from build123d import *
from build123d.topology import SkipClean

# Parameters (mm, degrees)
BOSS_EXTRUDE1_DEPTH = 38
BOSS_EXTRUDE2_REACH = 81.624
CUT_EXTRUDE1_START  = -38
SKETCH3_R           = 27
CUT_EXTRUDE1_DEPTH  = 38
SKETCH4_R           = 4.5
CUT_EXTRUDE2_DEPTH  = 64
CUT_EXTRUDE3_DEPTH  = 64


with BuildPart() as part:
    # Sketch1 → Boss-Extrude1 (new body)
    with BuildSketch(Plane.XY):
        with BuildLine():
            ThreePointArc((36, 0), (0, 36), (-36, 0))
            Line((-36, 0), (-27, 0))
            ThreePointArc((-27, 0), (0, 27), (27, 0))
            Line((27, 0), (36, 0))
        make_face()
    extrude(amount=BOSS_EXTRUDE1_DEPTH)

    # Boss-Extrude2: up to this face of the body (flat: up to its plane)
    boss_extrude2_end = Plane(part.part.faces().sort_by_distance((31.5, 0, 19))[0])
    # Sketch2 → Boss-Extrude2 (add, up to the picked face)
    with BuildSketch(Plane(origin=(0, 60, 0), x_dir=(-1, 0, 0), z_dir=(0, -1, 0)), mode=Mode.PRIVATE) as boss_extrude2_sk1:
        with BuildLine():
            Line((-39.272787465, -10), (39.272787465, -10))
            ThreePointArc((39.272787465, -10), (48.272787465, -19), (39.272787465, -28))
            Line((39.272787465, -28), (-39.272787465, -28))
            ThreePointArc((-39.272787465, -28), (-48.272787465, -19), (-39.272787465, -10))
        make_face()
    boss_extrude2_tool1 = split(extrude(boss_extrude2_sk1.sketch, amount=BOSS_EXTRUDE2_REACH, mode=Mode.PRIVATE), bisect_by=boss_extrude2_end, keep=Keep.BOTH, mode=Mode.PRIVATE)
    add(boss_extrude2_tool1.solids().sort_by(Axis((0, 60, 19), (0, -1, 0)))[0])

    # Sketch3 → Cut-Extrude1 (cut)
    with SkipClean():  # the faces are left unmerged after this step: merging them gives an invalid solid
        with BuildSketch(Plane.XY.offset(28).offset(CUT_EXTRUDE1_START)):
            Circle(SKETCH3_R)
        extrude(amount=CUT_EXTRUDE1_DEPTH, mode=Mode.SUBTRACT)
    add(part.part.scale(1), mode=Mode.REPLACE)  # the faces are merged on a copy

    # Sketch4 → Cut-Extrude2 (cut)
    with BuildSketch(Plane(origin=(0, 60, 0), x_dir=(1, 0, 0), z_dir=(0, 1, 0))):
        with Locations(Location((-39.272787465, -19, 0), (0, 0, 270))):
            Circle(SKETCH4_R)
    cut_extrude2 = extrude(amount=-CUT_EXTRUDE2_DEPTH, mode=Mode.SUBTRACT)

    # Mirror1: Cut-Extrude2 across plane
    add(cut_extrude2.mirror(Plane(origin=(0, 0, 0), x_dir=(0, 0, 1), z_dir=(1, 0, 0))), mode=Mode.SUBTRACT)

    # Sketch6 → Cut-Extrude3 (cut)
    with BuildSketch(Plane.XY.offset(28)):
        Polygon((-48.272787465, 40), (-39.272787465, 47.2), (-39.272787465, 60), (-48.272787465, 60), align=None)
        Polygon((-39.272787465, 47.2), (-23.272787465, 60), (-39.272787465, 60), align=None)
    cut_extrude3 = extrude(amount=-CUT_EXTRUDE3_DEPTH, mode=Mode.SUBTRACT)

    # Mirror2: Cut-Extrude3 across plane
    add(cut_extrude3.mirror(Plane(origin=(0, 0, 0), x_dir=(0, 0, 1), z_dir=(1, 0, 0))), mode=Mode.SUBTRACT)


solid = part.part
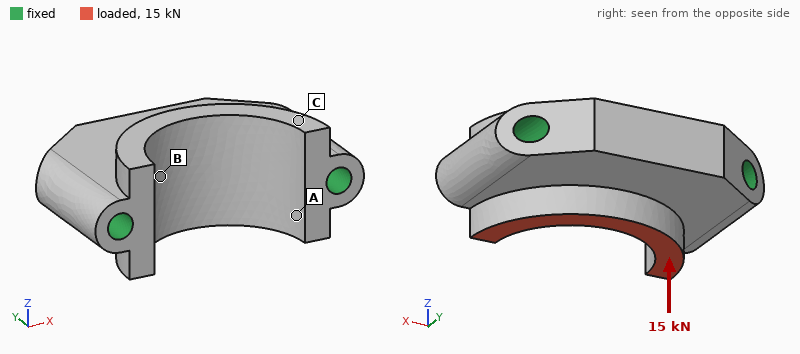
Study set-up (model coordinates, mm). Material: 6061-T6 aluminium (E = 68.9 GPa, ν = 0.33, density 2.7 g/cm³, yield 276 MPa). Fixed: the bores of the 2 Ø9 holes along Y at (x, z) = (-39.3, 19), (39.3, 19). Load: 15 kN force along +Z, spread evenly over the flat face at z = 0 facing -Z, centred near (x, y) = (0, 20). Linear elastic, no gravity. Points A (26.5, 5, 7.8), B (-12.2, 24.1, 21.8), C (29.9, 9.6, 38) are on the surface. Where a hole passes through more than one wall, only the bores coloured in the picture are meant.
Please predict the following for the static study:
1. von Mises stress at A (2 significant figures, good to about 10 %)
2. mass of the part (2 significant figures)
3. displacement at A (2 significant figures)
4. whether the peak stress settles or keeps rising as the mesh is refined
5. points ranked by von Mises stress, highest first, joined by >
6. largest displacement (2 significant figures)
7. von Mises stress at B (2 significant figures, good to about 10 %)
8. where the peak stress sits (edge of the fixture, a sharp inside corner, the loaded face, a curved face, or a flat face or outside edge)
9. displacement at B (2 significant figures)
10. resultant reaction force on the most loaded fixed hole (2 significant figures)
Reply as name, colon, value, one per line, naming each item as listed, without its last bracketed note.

von Mises stress at A: 17 MPa
mass of the part: 230 g
displacement at A: 9.0 µm
whether the peak stress settles or keeps rising as the mesh is refined: keeps rising
points ranked by von Mises stress, highest first, joined by >: A > B > C
largest displacement: 18 µm
von Mises stress at B: 11 MPa
where the peak stress sits: edge of the fixture
displacement at B: 13 µm
resultant reaction force on the most loaded fixed hole: 7.5 kN
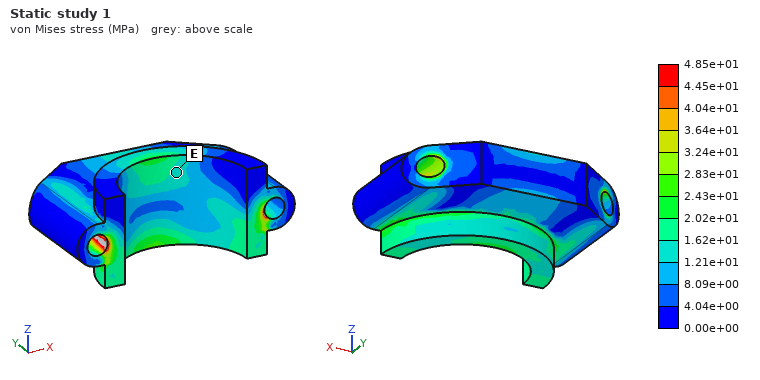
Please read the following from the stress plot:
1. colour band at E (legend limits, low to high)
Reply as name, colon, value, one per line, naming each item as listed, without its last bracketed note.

colour band at E: 1.21e+01 to 1.62e+01 MPa
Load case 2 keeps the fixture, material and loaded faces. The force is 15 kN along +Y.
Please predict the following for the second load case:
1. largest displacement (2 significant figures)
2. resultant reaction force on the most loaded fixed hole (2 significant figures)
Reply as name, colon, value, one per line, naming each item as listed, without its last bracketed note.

largest displacement: 46 µm
resultant reaction force on the most loaded fixed hole: 7.7 kN
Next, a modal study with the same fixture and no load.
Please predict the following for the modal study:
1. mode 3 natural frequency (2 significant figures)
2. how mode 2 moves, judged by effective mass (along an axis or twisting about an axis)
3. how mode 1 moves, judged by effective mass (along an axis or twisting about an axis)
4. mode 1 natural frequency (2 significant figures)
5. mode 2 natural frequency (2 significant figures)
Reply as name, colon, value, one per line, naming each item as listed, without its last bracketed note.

mode 3 natural frequency: 19 kHz
how mode 2 moves, judged by effective mass: along Y
how mode 1 moves, judged by effective mass: along Z
mode 1 natural frequency: 11 kHz
mode 2 natural frequency: 18 kHz
